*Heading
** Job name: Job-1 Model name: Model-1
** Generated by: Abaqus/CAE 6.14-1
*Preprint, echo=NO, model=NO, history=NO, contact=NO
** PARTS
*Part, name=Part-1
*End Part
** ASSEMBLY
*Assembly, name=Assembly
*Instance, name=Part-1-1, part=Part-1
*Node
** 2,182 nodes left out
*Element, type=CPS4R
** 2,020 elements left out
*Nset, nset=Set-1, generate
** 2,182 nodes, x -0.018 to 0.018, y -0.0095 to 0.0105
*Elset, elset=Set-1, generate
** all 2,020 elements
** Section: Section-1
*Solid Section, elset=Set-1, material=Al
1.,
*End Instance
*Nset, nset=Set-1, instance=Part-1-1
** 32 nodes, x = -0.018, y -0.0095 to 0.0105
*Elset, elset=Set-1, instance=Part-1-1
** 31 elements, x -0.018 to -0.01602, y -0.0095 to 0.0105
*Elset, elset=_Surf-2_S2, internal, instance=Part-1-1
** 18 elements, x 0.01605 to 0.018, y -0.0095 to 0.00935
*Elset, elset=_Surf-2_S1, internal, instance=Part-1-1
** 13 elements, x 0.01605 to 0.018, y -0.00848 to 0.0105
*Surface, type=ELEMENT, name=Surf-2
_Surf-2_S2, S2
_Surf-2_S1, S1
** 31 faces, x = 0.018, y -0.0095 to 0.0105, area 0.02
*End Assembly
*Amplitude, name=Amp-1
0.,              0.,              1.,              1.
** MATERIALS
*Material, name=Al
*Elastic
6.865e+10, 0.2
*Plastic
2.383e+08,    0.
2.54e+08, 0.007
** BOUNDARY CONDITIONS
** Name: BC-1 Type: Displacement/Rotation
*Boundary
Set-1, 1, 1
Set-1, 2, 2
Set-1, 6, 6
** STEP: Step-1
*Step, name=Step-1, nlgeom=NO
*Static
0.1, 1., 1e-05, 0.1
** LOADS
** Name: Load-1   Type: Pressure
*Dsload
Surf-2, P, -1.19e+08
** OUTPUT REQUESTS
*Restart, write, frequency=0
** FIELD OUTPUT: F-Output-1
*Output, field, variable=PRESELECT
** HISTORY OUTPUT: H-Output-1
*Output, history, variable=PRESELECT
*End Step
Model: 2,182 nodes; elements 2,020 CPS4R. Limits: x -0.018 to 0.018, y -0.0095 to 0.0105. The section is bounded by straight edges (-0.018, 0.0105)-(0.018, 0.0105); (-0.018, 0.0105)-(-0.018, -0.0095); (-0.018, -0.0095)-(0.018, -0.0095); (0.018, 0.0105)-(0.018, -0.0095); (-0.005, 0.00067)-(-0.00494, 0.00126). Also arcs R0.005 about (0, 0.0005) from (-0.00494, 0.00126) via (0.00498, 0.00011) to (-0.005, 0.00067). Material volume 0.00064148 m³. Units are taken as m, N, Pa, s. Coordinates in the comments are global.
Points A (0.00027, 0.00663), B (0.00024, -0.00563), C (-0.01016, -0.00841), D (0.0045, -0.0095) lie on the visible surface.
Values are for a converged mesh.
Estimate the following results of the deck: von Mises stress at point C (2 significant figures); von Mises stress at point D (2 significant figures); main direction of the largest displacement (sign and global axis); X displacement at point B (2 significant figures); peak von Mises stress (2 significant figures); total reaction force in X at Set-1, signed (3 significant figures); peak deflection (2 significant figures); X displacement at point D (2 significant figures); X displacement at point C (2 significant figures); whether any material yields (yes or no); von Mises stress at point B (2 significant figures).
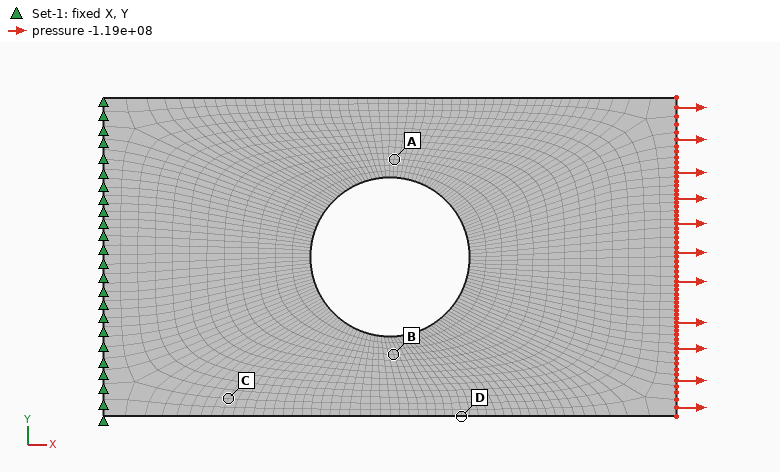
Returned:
1.9e+08 Pa
2.1e+08 Pa
+X
4.9e-05 m
2.6e+08 Pa
-2.38e+06 N
9.8e-05 m
5.6e-05 m
1.9e-05 m
yes
2.4e+08 Pa
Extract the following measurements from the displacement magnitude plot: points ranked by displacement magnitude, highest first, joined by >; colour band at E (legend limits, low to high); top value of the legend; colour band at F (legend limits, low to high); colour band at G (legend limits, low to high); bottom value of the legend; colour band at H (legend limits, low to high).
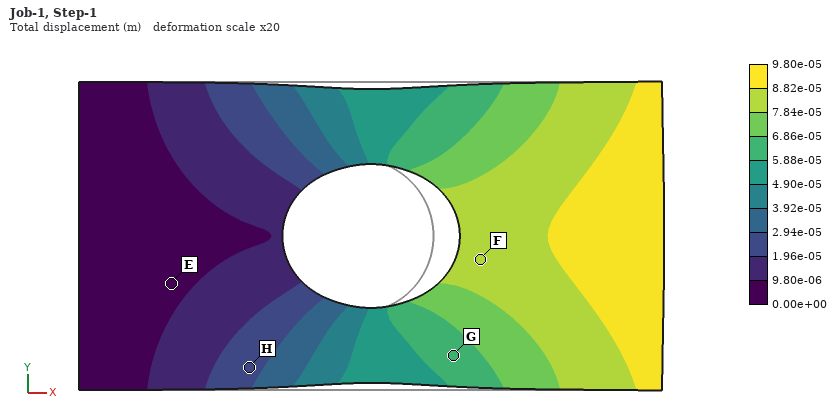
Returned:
F > G > H > E
0.00e+00 to 9.80e-06 m
9.80e-05 m
7.84e-05 to 8.82e-05 m
5.88e-05 to 6.86e-05 m
0.00e+00 m
1.96e-05 to 2.94e-05 m
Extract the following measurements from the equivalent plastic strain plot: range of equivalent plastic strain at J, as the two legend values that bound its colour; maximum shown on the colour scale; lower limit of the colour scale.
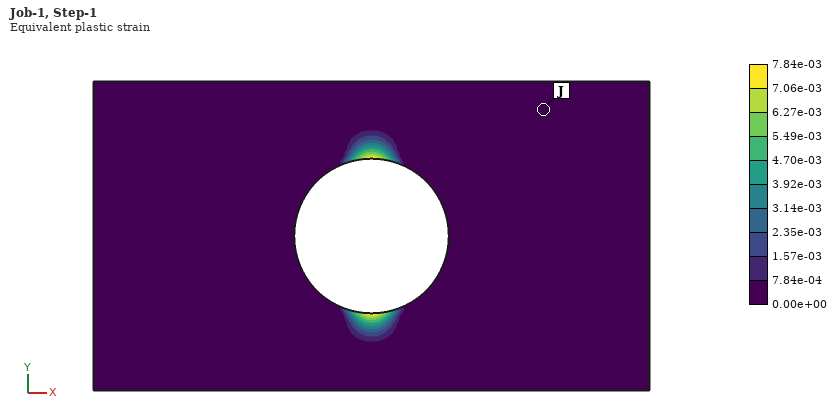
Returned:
0.00e+00 to 7.84e-04
7.84e-03
0.00e+00
